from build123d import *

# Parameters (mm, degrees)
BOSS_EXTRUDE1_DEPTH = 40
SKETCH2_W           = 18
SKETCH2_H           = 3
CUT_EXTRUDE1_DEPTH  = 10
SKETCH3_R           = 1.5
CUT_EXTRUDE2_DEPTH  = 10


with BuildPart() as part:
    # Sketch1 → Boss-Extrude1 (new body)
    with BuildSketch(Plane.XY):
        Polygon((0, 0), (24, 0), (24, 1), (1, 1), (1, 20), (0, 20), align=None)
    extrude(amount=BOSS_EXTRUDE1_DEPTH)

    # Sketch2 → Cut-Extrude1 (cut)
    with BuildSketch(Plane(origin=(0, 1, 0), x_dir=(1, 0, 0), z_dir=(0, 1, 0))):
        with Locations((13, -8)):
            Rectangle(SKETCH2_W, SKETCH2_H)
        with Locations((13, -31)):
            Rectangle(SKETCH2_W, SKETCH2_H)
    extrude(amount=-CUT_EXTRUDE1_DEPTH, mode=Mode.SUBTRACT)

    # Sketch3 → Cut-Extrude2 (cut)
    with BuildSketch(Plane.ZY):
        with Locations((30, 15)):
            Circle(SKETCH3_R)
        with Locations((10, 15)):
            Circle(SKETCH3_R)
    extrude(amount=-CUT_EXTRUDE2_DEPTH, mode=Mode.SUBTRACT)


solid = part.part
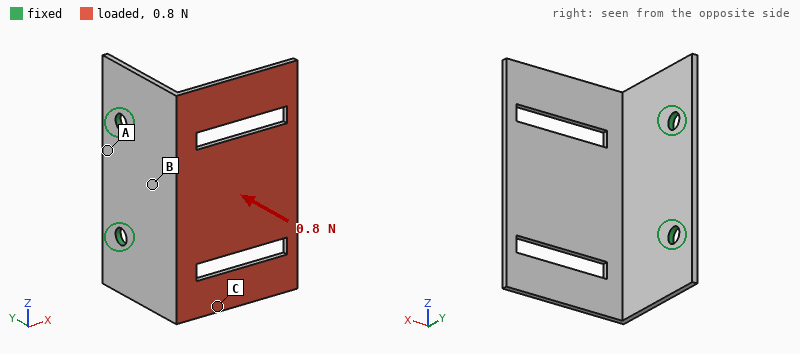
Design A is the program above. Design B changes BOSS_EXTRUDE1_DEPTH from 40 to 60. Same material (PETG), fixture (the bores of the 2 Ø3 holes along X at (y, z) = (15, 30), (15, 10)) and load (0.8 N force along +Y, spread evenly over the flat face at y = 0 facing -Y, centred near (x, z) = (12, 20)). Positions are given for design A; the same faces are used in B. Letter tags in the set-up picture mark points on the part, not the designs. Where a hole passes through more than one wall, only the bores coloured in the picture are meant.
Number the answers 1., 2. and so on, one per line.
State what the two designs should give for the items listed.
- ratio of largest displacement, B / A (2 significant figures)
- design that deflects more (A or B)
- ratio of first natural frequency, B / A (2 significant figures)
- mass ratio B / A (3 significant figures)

1. 0.91
2. A
3. 0.82
4. 1.54
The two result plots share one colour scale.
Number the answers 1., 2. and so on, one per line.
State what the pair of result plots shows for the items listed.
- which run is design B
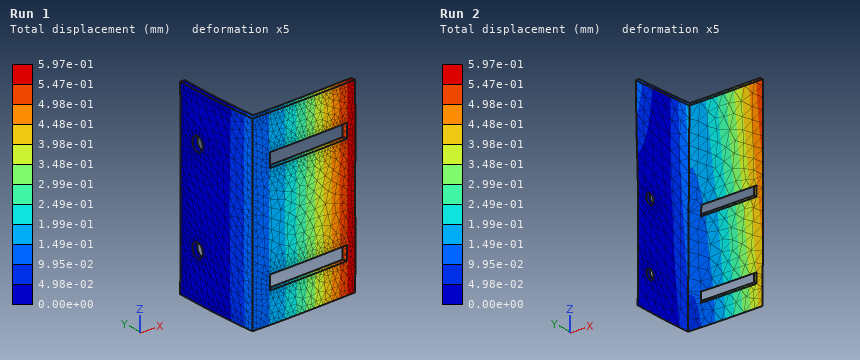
1. Run 2
